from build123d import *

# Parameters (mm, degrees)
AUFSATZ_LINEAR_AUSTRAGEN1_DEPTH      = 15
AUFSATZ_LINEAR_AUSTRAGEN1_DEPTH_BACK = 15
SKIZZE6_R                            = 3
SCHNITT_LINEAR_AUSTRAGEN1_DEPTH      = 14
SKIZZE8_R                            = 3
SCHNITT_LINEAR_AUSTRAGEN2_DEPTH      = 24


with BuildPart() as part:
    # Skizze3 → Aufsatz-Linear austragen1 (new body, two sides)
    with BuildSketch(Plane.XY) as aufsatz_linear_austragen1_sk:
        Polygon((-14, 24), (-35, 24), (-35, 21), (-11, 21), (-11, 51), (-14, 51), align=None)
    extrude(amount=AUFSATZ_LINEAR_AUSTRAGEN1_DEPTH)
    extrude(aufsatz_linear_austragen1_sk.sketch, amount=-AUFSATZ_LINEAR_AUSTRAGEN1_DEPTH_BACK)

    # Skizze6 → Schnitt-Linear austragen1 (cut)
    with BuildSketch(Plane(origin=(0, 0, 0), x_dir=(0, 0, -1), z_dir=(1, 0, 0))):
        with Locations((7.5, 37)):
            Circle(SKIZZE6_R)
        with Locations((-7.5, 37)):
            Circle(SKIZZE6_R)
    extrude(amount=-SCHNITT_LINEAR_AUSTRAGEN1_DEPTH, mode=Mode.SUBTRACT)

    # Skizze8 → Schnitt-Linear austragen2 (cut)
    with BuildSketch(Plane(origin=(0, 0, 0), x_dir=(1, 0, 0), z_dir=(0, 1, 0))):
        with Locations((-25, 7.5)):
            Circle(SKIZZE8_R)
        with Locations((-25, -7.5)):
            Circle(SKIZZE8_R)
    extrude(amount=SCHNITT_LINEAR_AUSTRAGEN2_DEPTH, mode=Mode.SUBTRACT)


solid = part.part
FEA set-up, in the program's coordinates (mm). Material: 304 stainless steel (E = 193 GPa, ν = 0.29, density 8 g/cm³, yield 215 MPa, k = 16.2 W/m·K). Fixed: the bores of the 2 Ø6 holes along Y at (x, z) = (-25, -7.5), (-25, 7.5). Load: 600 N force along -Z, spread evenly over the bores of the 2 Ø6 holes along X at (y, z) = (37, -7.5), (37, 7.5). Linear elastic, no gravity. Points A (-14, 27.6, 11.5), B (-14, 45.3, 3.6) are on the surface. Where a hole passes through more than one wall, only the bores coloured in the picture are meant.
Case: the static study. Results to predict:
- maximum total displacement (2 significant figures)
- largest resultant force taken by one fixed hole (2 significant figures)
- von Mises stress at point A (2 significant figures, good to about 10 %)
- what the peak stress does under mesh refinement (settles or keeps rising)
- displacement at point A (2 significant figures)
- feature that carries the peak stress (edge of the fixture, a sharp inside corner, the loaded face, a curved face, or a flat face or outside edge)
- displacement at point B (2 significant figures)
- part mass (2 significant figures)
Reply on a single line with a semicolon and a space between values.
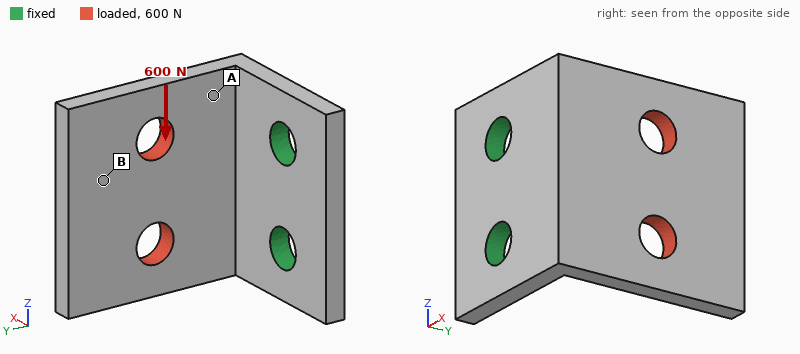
56 µm; 630 N; 51 MPa; keeps rising; 20 µm; edge of the fixture; 40 µm; 34 g
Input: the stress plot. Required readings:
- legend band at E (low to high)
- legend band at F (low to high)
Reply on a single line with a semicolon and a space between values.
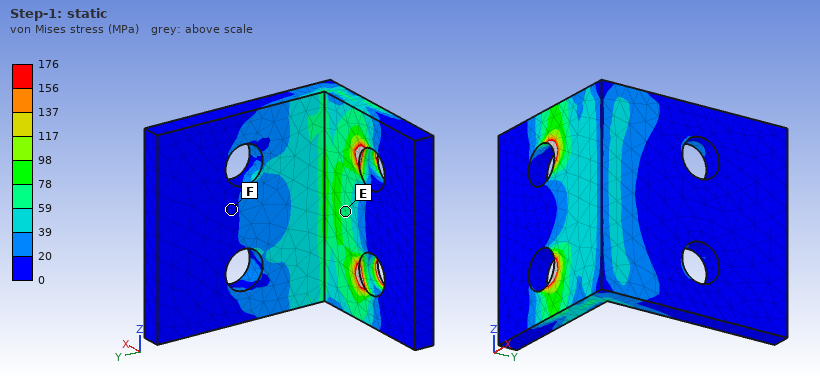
59 to 78 MPa; 0 to 20 MPa
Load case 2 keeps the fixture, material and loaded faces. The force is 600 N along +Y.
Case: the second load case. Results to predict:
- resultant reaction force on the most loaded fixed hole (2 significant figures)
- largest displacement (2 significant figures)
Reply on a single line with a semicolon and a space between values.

300 N; 75 µm
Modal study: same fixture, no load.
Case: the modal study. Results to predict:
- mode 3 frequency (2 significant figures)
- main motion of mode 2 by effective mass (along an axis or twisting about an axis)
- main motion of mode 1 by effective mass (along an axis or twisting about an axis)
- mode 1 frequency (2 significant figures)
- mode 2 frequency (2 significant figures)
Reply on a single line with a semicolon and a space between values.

6400 Hz; along Z; along X; 1900 Hz; 4200 Hz
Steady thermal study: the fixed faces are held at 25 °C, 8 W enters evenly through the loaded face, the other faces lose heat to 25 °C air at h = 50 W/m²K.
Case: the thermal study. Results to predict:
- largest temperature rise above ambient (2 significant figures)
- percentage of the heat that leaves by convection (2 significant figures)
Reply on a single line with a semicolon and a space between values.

68 K; 62 %
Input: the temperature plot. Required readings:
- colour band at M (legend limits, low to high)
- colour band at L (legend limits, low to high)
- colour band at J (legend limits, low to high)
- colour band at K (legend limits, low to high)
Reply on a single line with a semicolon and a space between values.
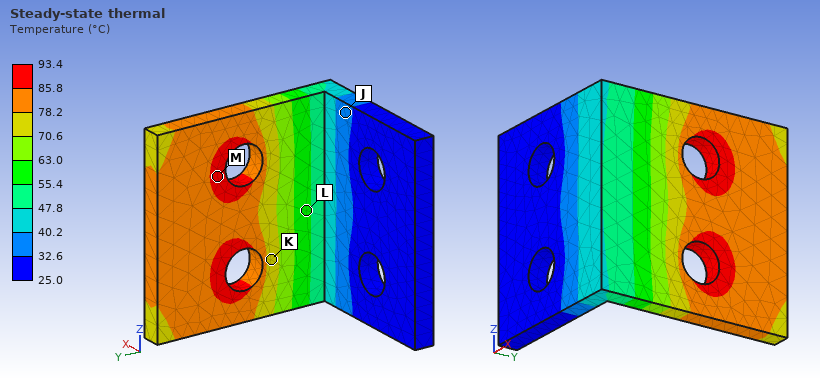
85.8 to 93.4 °C; 55.4 to 63.0 °C; 32.6 to 40.2 °C; 70.6 to 78.2 °C
